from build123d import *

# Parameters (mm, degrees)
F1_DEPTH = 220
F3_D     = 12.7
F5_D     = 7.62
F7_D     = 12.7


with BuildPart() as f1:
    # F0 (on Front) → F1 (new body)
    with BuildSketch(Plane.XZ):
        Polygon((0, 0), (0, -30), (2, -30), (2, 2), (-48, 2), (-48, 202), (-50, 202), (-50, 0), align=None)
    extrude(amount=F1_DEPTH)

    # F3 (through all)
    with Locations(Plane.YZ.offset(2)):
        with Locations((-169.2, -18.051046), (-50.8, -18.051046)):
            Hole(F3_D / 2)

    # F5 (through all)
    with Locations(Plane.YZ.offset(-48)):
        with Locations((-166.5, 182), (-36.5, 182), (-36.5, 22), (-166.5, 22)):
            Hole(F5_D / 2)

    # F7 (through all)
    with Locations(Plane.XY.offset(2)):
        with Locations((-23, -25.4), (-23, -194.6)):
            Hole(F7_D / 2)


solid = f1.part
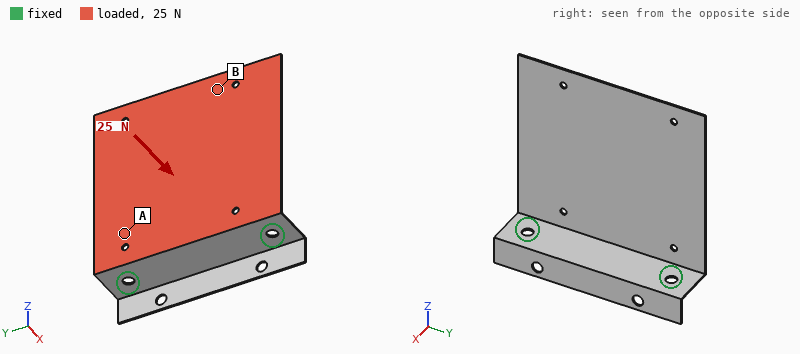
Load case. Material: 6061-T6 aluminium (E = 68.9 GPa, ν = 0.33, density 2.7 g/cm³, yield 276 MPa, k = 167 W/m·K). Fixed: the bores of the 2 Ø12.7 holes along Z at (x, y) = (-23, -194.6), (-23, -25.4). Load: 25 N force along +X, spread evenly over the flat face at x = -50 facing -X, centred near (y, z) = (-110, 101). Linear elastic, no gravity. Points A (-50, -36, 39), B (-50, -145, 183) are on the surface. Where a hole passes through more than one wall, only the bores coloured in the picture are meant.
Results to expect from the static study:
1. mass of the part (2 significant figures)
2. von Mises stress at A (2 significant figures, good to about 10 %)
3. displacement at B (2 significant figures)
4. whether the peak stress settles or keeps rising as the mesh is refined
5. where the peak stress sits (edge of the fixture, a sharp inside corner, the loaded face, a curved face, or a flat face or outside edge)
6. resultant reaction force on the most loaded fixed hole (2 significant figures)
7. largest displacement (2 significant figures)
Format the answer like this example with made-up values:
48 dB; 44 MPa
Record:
330 g; 9.6 MPa; 3.0 mm; keeps rising; edge of the fixture; 24 N; 3.5 mm
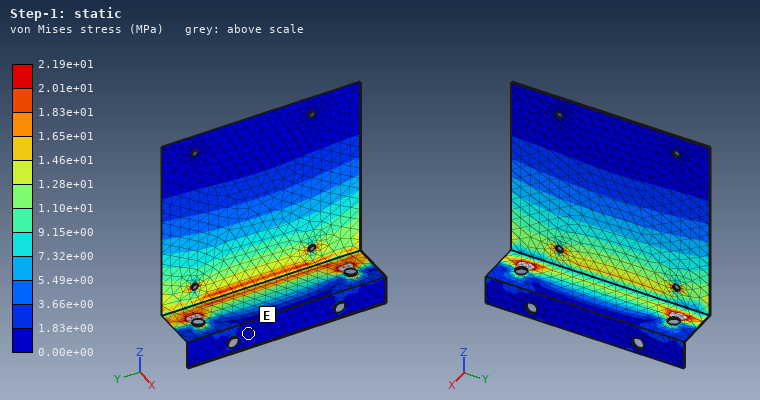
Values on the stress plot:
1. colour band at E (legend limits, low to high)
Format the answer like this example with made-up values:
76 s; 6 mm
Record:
0.00e+00 to 1.83e+00 MPa
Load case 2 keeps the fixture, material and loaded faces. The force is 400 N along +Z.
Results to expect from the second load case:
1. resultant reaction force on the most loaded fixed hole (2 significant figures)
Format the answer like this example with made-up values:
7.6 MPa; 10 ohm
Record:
210 N
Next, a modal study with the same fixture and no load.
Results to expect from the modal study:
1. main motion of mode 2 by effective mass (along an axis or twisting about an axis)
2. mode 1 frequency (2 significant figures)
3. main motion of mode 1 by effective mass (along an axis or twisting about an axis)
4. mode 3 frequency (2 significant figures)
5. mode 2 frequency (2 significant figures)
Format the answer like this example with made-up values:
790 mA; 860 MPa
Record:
twisting about Z; 34 Hz; along X; 220 Hz; 87 Hz
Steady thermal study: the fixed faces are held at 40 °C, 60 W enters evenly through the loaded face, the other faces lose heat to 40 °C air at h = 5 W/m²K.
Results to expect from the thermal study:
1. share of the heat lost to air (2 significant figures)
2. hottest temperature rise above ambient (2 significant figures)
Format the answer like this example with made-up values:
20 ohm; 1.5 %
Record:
31 %; 87 K
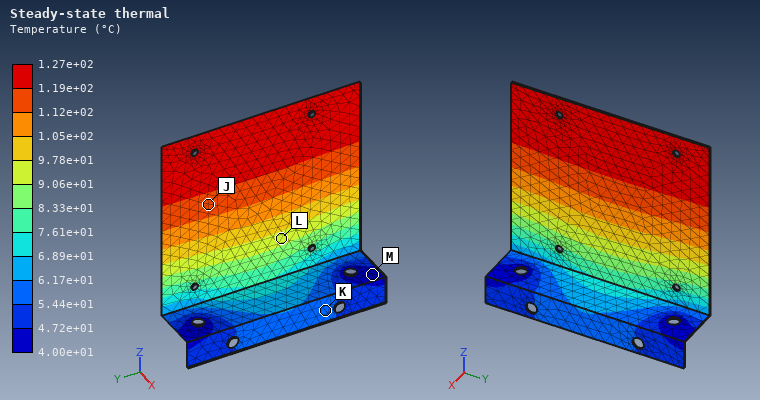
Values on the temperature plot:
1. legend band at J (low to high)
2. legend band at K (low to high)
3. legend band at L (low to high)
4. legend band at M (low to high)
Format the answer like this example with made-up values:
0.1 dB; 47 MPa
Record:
1.12e+02 to 1.19e+02 °C; 5.44e+01 to 6.17e+01 °C; 9.06e+01 to 9.78e+01 °C; 4.00e+01 to 4.72e+01 °C
